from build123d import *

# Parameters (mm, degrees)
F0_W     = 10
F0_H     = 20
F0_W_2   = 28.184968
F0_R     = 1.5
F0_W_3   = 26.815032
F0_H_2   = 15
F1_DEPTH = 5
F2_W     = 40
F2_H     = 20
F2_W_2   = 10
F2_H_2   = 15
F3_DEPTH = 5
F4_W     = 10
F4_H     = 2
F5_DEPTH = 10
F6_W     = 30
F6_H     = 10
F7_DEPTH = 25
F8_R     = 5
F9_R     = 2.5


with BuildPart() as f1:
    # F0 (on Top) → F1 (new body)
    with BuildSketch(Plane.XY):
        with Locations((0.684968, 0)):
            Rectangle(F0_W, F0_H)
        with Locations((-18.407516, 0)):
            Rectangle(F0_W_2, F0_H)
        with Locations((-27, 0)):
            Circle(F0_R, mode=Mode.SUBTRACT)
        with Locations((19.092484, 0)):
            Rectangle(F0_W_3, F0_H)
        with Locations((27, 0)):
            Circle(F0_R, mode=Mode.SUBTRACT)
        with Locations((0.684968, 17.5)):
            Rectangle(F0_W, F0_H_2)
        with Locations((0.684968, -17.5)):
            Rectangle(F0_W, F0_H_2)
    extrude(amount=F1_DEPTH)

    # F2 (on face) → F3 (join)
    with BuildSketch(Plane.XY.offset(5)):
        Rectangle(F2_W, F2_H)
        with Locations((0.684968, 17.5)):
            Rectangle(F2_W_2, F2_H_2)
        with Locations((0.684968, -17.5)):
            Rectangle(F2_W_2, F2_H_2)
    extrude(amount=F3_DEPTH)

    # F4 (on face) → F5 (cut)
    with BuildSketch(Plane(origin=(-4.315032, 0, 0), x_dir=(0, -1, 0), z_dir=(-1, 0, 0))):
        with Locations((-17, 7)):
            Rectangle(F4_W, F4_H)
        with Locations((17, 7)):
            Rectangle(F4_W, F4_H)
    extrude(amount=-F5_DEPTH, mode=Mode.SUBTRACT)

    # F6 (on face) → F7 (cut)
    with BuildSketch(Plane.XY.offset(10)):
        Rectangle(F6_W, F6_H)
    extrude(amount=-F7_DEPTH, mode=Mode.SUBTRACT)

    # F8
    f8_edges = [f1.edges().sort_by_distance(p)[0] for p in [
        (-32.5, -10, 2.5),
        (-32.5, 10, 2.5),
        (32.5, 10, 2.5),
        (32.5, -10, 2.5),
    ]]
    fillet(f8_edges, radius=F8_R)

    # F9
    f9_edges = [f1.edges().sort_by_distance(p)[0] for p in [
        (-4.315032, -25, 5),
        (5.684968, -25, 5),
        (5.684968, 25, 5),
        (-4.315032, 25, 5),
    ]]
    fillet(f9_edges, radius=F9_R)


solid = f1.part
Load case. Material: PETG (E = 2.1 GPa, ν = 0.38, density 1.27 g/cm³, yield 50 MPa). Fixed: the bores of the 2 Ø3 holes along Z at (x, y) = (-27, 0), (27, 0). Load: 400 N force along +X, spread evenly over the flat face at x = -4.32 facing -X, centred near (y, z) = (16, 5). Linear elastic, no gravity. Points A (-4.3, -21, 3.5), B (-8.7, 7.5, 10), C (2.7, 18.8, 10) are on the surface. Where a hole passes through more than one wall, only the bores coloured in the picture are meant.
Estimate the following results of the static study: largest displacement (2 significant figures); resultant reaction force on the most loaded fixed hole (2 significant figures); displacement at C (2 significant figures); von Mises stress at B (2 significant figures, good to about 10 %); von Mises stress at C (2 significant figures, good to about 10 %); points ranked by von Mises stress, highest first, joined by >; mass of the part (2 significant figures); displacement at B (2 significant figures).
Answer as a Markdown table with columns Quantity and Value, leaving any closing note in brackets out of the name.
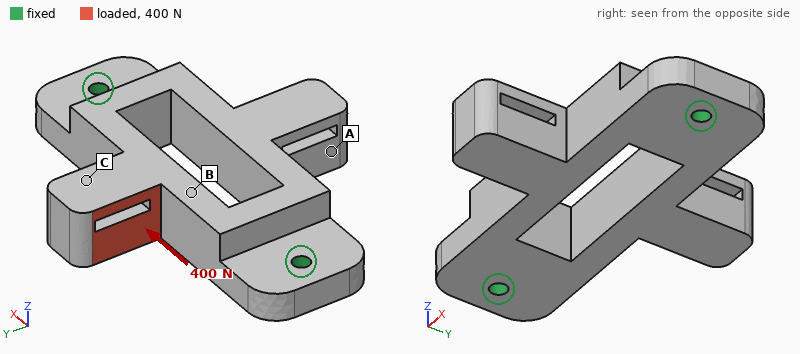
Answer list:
| Quantity | Value |
|---|---|
| largest displacement | 0.56 mm |
| resultant reaction force on the most loaded fixed hole | 240 N |
| displacement at C | 0.34 mm |
| von Mises stress at B | 7.5 MPa |
| von Mises stress at C | 4.6 MPa |
| points ranked by von Mises stress, highest first, joined by > | B > C > A |
| mass of the part | 13 g |
| displacement at B | 0.13 mm |
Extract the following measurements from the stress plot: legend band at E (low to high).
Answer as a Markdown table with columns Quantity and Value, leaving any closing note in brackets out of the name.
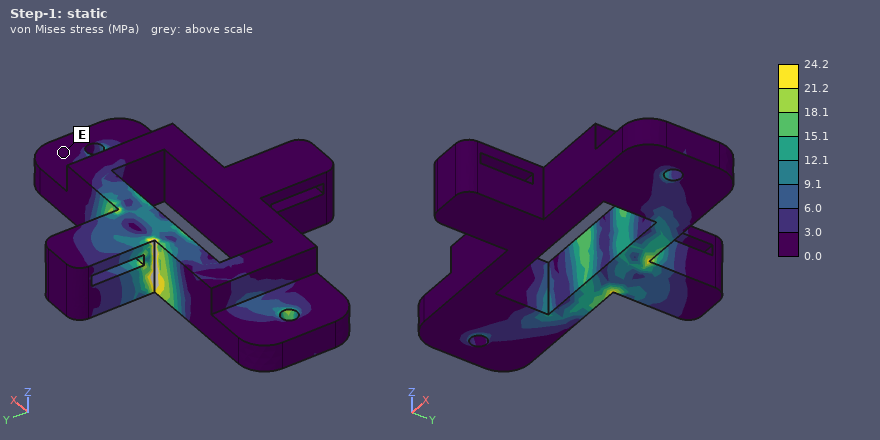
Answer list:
| Quantity | Value |
|---|---|
| legend band at E | 0.0 to 3.0 MPa |
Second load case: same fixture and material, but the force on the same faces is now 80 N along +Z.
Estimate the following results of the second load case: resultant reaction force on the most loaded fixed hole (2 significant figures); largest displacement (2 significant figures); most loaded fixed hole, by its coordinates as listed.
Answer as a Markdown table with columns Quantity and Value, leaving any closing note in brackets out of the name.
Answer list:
| Quantity | Value |
|---|---|
| resultant reaction force on the most loaded fixed hole | 70 N |
| largest displacement | 0.81 mm |
| most loaded fixed hole, by its coordinates as listed | (-27, 0) |
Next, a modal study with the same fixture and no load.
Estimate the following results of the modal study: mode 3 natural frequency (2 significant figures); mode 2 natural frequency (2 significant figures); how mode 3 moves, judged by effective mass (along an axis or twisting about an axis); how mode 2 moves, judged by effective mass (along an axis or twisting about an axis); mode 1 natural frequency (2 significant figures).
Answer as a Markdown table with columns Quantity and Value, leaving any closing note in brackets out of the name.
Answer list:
| Quantity | Value |
|---|---|
| mode 3 natural frequency | 2600 Hz |
| mode 2 natural frequency | 1500 Hz |
| how mode 3 moves, judged by effective mass | along Y |
| how mode 2 moves, judged by effective mass | along Z |
| mode 1 natural frequency | 1100 Hz |
